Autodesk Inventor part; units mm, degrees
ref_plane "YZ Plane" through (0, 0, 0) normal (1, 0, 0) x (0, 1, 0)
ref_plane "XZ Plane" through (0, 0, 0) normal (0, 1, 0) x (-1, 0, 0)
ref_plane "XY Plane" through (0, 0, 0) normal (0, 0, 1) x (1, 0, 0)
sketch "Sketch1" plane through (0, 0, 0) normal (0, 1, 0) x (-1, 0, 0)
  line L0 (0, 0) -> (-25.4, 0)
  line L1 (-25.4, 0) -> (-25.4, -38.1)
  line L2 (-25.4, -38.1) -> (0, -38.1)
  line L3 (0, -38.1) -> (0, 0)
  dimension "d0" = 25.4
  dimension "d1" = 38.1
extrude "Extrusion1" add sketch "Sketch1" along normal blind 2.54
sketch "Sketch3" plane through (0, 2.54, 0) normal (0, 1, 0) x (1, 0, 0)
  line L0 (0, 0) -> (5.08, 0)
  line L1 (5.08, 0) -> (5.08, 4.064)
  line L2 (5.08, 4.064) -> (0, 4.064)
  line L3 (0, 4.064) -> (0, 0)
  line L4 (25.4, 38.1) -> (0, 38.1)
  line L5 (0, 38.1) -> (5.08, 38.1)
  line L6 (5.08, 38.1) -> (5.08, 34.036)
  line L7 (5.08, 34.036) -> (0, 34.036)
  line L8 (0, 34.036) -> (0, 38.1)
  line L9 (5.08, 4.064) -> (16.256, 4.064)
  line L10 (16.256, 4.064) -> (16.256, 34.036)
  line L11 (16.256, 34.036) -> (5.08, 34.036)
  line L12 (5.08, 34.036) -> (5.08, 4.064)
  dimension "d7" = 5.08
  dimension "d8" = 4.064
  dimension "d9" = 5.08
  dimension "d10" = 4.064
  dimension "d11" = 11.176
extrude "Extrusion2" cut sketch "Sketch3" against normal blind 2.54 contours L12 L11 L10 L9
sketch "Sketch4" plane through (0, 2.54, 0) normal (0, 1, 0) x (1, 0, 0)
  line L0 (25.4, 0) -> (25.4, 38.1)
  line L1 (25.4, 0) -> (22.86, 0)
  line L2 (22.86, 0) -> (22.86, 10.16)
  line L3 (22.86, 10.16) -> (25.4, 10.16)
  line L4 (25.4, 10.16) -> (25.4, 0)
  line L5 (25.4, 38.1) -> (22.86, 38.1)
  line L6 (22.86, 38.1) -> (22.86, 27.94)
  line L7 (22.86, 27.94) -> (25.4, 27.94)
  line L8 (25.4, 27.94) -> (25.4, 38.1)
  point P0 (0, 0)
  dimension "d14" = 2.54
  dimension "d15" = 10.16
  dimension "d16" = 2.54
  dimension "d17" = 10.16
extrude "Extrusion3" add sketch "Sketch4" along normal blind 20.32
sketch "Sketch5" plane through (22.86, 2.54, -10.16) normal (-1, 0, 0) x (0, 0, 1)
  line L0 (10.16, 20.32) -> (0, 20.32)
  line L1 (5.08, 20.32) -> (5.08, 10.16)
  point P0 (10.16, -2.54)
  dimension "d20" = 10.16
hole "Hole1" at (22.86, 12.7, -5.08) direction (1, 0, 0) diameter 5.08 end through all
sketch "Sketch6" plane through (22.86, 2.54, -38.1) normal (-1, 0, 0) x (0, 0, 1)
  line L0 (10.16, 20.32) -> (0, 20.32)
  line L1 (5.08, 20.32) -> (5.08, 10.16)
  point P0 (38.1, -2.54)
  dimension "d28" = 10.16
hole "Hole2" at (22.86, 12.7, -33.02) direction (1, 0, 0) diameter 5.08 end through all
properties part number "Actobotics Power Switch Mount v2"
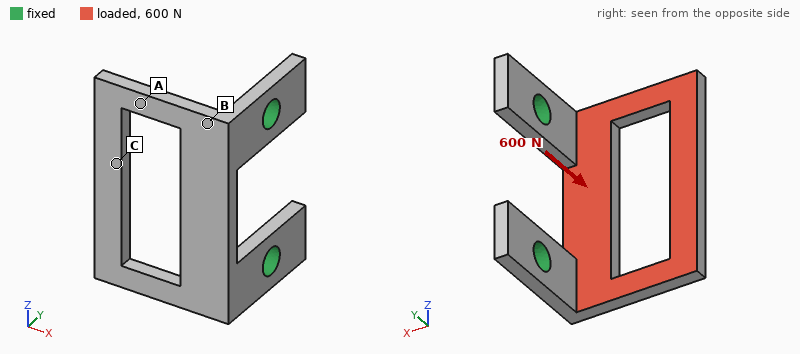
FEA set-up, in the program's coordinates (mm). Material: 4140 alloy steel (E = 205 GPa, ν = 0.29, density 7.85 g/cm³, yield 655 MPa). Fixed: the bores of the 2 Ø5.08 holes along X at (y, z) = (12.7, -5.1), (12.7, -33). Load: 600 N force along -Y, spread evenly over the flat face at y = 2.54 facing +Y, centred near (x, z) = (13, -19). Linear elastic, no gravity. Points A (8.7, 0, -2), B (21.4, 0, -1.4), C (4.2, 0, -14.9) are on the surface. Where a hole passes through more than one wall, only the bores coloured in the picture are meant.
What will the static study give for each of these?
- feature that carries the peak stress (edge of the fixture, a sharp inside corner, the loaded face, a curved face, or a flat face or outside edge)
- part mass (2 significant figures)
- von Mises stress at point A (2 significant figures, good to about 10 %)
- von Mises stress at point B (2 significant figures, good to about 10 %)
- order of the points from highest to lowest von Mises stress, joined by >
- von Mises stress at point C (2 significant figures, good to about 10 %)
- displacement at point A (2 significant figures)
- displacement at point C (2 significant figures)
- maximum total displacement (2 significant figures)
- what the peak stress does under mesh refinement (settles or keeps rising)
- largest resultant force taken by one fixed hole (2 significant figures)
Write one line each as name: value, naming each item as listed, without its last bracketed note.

feature that carries the peak stress: a sharp inside corner
part mass: 20 g
von Mises stress at point A: 160 MPa
von Mises stress at point B: 260 MPa
order of the points from highest to lowest von Mises stress, joined by >: B > A > C
von Mises stress at point C: 78 MPa
displacement at point A: 0.29 mm
displacement at point C: 0.44 mm
maximum total displacement: 0.56 mm
what the peak stress does under mesh refinement: keeps rising
largest resultant force taken by one fixed hole: 300 N
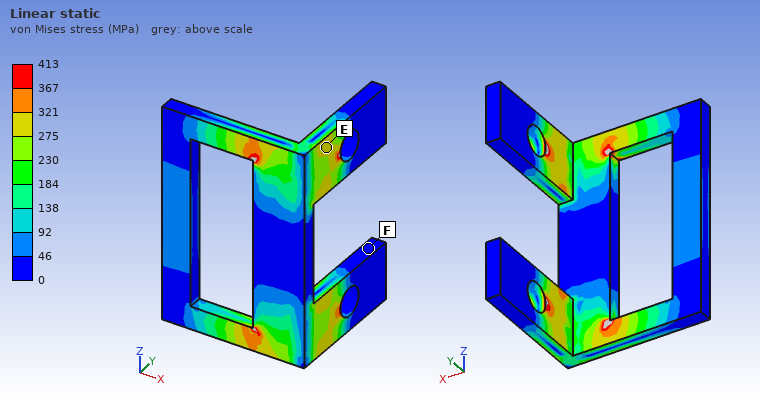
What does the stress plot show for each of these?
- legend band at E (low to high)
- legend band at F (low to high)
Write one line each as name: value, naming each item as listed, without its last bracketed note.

legend band at E: 275 to 321 MPa
legend band at F: 0 to 46 MPa
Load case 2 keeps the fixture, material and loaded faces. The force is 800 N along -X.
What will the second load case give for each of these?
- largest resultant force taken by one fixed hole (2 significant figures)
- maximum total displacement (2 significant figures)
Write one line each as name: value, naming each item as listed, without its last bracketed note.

largest resultant force taken by one fixed hole: 400 N
maximum total displacement: 82 µm
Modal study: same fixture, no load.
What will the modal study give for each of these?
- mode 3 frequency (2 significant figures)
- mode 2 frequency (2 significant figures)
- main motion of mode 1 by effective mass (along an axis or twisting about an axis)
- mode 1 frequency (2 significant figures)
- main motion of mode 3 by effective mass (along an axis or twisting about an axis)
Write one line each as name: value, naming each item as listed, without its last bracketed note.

mode 3 frequency: 5700 Hz
mode 2 frequency: 4000 Hz
main motion of mode 1 by effective mass: along Y
mode 1 frequency: 1800 Hz
main motion of mode 3 by effective mass: along Z
